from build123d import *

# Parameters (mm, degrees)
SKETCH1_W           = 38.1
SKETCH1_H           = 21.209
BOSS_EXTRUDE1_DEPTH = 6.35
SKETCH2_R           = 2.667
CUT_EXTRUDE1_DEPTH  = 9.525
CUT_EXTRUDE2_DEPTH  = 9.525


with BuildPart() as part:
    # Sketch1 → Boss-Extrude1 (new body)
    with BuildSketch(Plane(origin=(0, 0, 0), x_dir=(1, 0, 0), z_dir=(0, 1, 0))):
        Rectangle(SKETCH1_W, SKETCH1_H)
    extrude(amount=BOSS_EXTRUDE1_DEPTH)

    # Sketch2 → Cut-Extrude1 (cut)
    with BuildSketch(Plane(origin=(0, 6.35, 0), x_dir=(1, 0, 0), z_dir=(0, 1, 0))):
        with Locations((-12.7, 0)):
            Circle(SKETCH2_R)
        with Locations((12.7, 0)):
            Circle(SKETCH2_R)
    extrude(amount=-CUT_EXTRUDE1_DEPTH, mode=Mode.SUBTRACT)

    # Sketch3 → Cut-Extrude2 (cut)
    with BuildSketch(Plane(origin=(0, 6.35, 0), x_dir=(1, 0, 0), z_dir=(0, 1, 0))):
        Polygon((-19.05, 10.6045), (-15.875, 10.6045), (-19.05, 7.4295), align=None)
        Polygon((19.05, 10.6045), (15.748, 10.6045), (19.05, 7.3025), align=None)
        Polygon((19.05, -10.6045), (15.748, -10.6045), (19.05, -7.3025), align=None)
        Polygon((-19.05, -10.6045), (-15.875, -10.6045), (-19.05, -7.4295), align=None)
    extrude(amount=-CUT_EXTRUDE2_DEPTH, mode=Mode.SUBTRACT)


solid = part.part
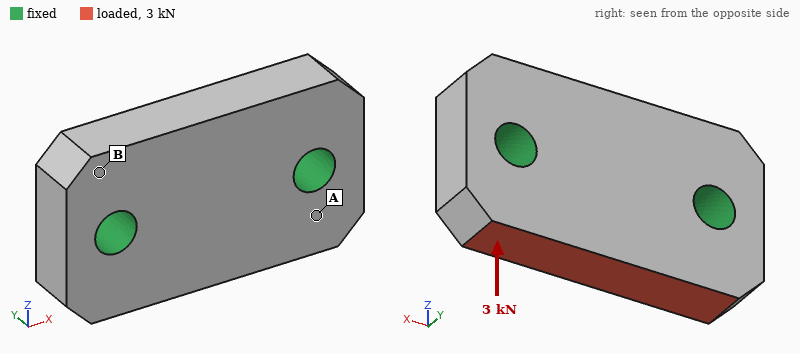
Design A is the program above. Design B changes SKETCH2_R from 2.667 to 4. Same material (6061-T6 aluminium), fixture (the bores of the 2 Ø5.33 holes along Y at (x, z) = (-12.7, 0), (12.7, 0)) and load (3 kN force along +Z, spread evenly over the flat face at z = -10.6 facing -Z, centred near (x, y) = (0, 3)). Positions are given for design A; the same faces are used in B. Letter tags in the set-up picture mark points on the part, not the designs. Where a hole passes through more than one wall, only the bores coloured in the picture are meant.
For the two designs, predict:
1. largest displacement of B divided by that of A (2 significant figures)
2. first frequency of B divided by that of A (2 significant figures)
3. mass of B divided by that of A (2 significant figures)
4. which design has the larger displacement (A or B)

0.81
1.3
0.92
A
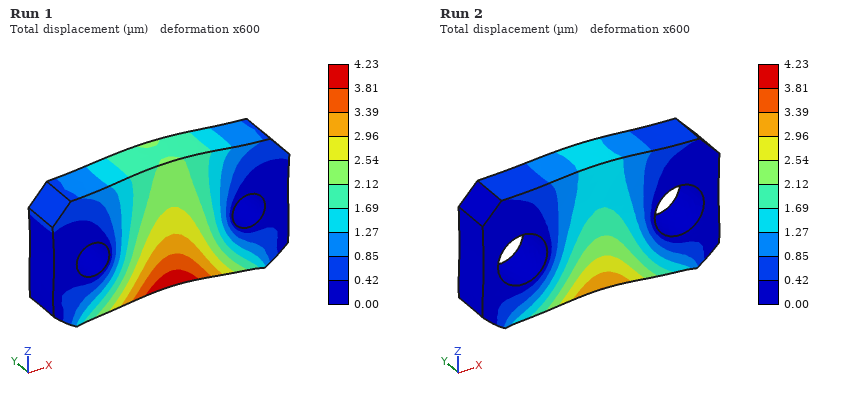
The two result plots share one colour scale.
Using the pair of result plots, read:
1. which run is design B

Run 2
